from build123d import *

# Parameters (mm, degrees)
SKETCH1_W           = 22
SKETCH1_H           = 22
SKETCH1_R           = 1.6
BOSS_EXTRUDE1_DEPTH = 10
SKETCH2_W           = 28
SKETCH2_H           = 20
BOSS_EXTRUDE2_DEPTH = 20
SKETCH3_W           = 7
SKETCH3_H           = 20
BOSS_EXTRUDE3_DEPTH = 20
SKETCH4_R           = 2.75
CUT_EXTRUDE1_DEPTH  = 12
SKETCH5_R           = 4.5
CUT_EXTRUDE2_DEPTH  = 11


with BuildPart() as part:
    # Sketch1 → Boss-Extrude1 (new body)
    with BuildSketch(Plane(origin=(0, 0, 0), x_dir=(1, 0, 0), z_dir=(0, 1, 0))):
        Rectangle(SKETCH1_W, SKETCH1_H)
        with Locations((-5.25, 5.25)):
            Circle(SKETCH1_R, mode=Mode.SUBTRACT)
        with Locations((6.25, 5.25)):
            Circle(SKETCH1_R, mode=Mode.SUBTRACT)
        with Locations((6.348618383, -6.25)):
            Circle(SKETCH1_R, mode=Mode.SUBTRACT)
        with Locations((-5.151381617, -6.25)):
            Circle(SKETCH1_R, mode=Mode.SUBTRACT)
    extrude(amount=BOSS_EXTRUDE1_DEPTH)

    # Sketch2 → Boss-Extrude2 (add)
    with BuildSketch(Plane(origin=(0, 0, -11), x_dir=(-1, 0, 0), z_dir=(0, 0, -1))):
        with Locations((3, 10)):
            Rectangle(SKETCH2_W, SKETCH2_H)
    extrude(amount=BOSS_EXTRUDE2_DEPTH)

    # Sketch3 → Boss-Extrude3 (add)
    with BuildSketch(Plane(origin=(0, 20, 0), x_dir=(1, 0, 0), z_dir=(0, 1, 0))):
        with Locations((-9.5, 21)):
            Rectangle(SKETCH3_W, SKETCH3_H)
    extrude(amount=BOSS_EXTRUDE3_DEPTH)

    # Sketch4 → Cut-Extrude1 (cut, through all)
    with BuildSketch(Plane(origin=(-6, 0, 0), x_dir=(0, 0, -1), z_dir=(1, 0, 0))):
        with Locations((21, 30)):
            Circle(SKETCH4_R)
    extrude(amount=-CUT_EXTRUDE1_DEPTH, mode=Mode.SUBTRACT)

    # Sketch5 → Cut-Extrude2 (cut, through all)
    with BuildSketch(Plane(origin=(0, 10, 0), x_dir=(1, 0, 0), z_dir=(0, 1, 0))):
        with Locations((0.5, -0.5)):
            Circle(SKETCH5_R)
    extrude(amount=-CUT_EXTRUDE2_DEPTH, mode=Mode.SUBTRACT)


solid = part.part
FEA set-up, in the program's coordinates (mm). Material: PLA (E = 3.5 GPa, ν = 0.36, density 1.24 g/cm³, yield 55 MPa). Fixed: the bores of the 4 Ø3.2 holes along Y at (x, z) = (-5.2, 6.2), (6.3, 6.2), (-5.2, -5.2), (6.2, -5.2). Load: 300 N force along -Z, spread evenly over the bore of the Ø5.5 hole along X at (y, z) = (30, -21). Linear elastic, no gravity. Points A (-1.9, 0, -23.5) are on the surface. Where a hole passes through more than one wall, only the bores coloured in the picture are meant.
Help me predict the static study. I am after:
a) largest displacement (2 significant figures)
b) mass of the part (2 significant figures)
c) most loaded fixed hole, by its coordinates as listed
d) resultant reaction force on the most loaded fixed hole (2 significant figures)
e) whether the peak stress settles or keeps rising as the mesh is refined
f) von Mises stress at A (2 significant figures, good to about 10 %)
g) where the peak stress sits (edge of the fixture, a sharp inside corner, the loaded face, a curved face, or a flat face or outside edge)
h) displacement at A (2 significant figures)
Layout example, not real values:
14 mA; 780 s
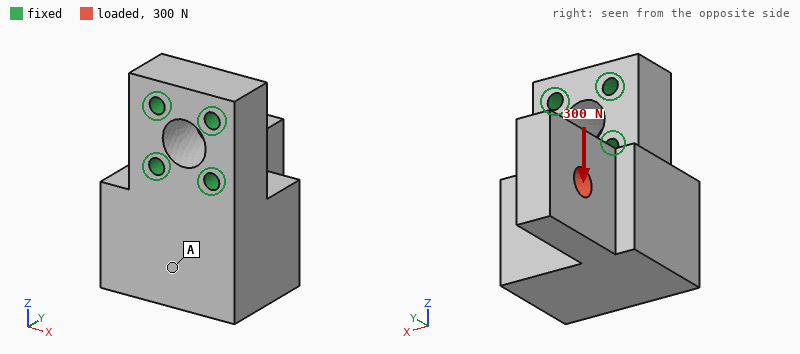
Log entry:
0.62 mm; 22 g; (-5.2, -5.2); 320 N; keeps rising; 3.2 MPa; edge of the fixture; 0.18 mm
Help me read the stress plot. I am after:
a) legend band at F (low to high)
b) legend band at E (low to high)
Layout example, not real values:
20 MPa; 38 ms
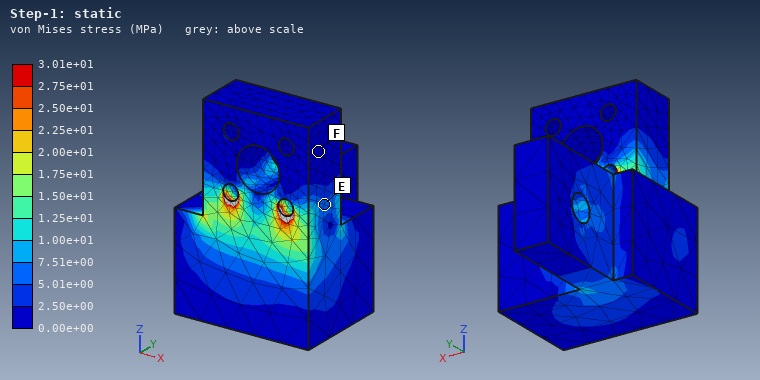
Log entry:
0.00e+00 to 2.50e+00 MPa; 5.01e+00 to 7.51e+00 MPa
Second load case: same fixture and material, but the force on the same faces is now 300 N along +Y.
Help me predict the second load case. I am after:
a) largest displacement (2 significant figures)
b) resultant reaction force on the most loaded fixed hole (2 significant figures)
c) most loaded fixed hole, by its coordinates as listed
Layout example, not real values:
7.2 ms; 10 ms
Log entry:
0.28 mm; 320 N; (-5.2, -5.2)
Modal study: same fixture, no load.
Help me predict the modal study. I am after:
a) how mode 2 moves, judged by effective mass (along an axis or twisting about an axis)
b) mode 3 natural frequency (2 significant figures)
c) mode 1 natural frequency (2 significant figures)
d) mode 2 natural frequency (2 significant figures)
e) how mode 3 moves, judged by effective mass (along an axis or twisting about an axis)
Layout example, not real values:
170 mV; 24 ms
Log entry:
along X; 3800 Hz; 1600 Hz; 2200 Hz; along X
